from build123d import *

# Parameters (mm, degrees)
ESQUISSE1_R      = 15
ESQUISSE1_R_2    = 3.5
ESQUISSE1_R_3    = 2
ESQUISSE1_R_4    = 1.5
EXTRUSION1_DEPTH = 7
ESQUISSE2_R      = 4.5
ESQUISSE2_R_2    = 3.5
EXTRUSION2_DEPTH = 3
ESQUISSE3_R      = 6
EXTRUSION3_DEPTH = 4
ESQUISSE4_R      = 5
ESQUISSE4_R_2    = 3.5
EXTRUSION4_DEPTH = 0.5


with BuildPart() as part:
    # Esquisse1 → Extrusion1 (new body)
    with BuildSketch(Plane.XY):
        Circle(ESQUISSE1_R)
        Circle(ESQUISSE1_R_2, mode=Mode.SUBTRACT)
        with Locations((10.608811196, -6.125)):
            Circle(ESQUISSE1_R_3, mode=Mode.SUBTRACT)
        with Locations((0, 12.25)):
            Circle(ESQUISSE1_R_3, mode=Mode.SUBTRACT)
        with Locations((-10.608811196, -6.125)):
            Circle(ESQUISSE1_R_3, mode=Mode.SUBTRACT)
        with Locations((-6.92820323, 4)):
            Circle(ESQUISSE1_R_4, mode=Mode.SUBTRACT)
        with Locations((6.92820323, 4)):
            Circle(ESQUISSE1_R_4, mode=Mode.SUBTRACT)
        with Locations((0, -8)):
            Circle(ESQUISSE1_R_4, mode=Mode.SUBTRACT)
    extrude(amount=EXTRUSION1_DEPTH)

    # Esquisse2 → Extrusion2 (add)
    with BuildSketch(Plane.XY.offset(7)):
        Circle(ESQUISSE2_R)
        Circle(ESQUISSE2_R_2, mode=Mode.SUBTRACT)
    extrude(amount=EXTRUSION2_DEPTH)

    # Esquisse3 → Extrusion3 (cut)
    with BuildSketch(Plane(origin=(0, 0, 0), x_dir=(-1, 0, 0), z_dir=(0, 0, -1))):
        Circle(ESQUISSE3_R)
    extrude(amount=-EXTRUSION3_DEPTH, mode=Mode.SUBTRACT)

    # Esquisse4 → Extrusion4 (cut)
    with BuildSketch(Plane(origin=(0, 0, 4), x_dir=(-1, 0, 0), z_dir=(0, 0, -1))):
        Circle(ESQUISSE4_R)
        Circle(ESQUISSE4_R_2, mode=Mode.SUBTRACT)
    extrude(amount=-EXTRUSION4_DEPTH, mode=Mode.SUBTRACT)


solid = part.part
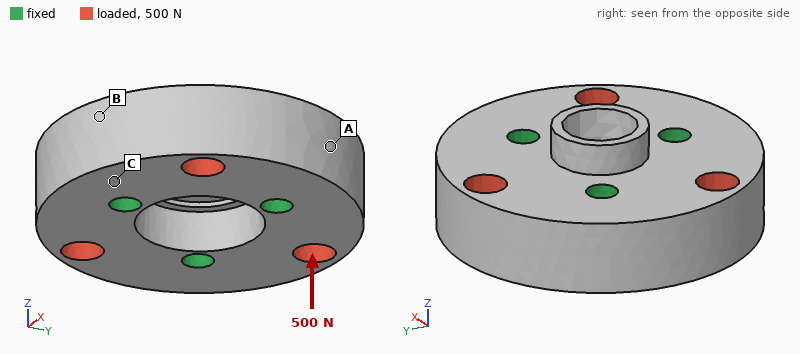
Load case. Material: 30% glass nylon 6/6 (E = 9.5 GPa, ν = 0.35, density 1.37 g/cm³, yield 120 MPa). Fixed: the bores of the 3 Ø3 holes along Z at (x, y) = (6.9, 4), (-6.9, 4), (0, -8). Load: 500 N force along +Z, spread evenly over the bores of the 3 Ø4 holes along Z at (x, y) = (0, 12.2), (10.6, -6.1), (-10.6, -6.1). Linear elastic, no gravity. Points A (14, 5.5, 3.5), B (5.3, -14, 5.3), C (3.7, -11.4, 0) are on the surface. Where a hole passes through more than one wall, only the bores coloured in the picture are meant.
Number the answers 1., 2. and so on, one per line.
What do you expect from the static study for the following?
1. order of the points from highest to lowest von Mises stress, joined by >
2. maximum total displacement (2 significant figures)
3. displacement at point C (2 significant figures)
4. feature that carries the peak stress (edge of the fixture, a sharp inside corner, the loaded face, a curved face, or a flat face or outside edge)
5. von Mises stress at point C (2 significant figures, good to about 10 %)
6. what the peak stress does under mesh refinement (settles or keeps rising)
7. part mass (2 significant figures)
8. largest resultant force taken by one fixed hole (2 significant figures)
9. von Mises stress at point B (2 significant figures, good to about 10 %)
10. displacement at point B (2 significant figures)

1. C > B > A
2. 18 µm
3. 3.7 µm
4. a sharp inside corner
5. 5.4 MPa
6. keeps rising
7. 5.5 g
8. 170 N
9. 2.8 MPa
10. 4.0 µm
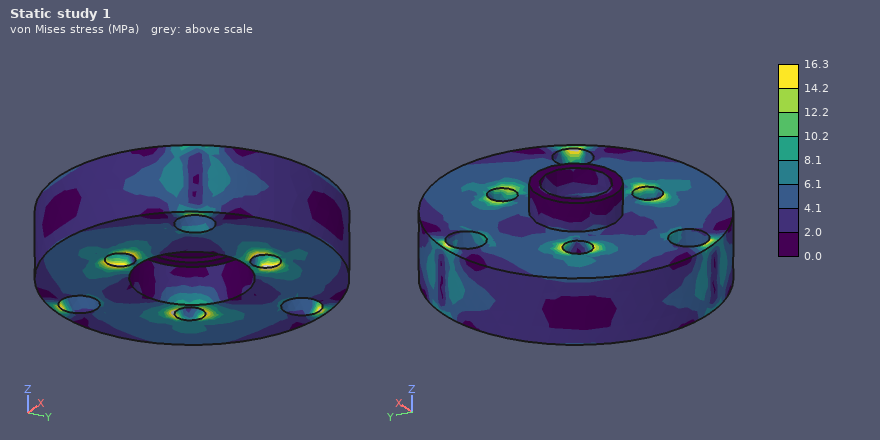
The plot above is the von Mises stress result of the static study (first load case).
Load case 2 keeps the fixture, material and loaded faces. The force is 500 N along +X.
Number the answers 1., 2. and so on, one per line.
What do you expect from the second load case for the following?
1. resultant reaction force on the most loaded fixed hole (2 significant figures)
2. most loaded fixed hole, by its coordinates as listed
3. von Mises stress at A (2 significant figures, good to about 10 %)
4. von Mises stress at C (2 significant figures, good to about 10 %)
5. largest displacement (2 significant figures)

1. 240 N
2. (0, -8)
3. 1.9 MPa
4. 1.0 MPa
5. 6.1 µm
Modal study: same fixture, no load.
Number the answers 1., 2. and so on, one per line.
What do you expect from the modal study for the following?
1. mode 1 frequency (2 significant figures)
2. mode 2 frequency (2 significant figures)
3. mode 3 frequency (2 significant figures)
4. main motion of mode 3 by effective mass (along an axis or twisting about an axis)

1. 22 kHz
2. 22 kHz
3. 25 kHz
4. along Z
